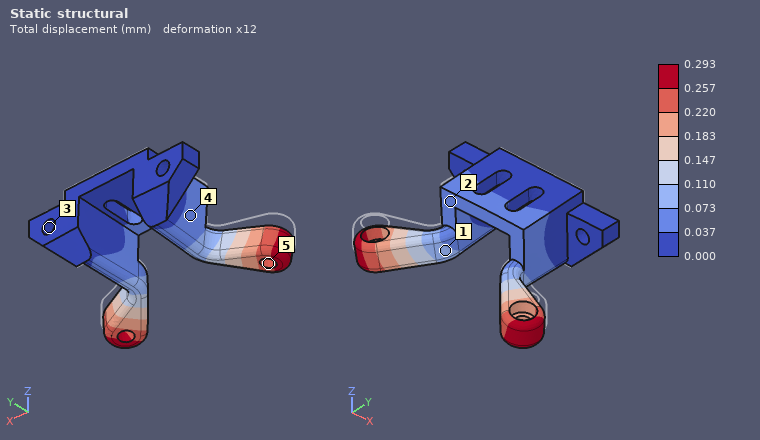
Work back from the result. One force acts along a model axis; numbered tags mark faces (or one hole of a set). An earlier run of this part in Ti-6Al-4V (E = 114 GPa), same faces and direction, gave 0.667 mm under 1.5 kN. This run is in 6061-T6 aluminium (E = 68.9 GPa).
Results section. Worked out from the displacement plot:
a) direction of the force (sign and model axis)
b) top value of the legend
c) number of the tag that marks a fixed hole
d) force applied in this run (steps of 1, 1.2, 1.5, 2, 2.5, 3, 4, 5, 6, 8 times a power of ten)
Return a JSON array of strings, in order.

["-Z", "0.293 mm", "3", "400 N"]
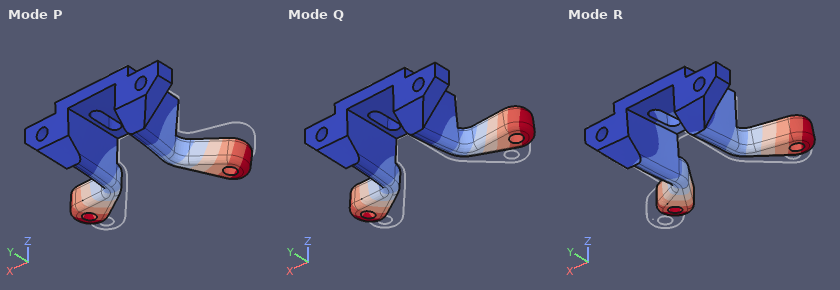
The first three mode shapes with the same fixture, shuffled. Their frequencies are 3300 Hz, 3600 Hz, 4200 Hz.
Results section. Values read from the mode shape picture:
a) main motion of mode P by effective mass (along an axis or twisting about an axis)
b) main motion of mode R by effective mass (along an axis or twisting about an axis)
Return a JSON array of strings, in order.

["along X", "along Z"]
